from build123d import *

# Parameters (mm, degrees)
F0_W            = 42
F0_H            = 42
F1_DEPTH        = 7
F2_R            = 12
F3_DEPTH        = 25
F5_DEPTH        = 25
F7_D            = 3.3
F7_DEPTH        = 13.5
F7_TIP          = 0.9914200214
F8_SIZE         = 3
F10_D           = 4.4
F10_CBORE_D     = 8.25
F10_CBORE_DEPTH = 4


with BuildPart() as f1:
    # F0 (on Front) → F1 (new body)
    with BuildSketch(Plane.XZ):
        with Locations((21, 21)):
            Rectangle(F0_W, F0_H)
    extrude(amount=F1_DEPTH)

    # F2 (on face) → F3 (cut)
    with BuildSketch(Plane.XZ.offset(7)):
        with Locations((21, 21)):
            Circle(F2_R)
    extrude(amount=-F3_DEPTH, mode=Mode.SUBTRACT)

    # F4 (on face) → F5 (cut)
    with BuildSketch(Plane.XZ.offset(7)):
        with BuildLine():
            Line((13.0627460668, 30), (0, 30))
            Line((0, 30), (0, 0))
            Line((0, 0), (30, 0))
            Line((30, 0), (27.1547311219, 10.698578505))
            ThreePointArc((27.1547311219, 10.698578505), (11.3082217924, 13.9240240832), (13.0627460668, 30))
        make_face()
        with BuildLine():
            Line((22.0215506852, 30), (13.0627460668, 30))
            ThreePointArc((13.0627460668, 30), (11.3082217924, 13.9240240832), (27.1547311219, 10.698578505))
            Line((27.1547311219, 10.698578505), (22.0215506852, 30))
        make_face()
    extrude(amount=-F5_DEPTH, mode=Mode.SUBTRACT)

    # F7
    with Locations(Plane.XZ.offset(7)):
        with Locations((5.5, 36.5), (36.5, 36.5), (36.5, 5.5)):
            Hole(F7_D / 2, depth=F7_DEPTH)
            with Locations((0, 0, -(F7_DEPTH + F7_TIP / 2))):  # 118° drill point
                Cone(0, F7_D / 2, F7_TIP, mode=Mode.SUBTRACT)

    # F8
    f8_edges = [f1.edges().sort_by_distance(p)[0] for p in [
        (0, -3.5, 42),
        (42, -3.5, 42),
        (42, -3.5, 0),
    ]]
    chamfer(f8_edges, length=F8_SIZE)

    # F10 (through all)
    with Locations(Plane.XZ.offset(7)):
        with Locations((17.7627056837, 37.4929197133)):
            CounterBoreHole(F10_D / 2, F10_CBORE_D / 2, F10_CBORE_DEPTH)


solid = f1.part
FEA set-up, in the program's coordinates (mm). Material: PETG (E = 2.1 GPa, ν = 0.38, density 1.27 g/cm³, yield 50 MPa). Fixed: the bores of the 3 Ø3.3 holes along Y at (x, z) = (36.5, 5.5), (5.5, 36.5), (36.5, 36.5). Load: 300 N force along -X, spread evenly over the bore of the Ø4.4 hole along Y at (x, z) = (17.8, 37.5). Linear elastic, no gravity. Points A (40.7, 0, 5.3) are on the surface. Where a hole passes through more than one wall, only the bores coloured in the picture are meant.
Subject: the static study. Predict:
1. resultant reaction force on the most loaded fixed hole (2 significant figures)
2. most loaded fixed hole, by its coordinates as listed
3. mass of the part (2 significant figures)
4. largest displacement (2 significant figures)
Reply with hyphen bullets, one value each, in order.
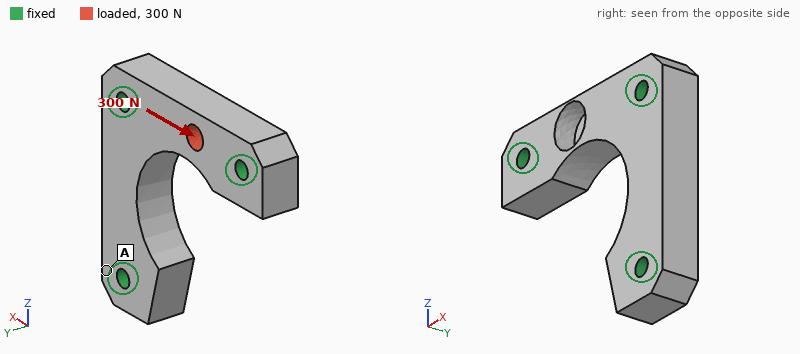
- 170 N
- (5.5, 36.5)
- 6.6 g
- 30 µm
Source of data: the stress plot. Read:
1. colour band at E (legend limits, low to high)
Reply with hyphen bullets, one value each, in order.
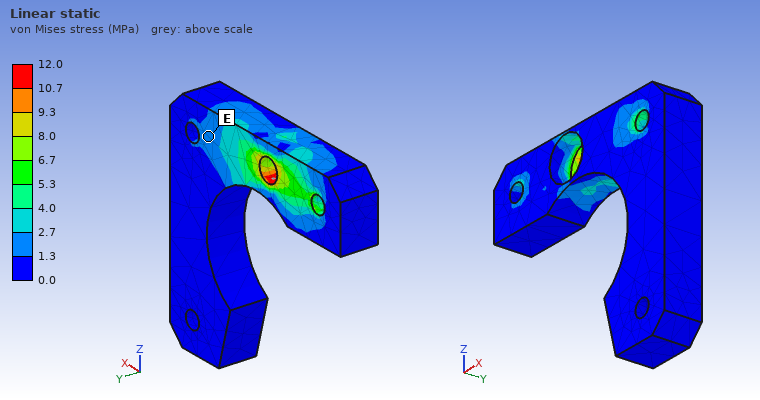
- 1.3 to 2.7 MPa
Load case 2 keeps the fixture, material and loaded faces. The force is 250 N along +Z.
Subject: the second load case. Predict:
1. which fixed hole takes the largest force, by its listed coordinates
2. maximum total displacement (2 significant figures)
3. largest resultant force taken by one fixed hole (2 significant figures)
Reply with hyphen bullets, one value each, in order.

- (5.5, 36.5)
- 0.12 mm
- 140 N
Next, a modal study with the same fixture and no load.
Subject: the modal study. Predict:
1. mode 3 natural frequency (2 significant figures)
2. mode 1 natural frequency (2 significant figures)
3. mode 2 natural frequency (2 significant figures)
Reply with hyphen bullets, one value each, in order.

- 7900 Hz
- 7000 Hz
- 7700 Hz
